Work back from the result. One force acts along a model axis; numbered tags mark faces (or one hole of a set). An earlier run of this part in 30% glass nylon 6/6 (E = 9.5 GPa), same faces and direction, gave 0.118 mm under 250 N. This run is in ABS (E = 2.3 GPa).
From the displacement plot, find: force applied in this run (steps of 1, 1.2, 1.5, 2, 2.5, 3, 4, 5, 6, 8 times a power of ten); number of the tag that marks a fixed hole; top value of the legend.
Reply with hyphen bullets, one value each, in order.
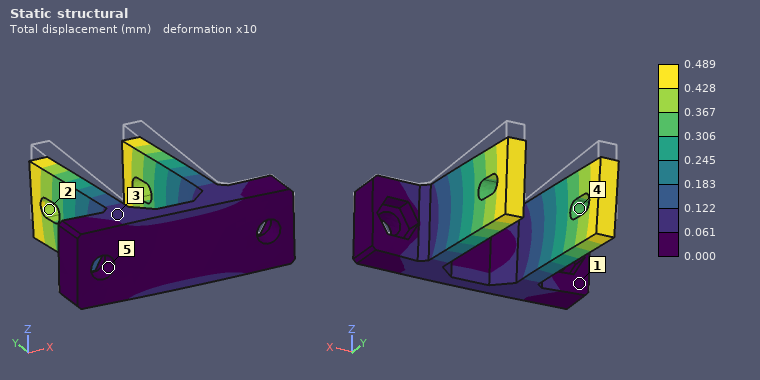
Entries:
- 250 N
- 5
- 0.489 mm
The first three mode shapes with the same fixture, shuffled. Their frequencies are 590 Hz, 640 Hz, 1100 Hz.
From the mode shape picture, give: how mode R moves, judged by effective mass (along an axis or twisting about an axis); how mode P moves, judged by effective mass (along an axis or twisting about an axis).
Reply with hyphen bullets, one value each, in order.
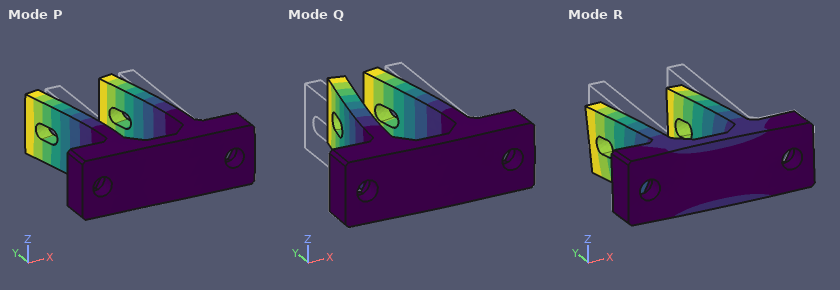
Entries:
- along Z
- along X
